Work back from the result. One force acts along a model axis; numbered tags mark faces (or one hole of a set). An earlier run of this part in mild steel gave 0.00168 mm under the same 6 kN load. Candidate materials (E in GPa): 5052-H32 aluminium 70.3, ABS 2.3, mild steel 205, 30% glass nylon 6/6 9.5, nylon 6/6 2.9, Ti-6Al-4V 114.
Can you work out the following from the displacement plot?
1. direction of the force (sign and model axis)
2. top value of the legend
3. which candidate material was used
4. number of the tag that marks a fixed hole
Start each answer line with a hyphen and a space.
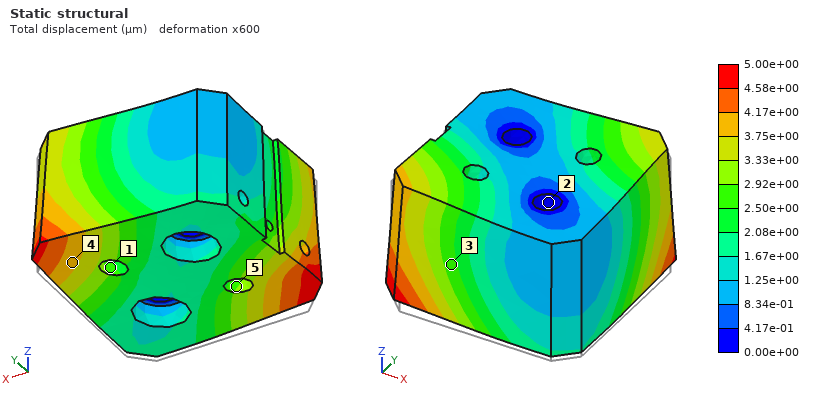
- +Z
- 5.00e+00 µm
- 5052-H32 aluminium
- 2
